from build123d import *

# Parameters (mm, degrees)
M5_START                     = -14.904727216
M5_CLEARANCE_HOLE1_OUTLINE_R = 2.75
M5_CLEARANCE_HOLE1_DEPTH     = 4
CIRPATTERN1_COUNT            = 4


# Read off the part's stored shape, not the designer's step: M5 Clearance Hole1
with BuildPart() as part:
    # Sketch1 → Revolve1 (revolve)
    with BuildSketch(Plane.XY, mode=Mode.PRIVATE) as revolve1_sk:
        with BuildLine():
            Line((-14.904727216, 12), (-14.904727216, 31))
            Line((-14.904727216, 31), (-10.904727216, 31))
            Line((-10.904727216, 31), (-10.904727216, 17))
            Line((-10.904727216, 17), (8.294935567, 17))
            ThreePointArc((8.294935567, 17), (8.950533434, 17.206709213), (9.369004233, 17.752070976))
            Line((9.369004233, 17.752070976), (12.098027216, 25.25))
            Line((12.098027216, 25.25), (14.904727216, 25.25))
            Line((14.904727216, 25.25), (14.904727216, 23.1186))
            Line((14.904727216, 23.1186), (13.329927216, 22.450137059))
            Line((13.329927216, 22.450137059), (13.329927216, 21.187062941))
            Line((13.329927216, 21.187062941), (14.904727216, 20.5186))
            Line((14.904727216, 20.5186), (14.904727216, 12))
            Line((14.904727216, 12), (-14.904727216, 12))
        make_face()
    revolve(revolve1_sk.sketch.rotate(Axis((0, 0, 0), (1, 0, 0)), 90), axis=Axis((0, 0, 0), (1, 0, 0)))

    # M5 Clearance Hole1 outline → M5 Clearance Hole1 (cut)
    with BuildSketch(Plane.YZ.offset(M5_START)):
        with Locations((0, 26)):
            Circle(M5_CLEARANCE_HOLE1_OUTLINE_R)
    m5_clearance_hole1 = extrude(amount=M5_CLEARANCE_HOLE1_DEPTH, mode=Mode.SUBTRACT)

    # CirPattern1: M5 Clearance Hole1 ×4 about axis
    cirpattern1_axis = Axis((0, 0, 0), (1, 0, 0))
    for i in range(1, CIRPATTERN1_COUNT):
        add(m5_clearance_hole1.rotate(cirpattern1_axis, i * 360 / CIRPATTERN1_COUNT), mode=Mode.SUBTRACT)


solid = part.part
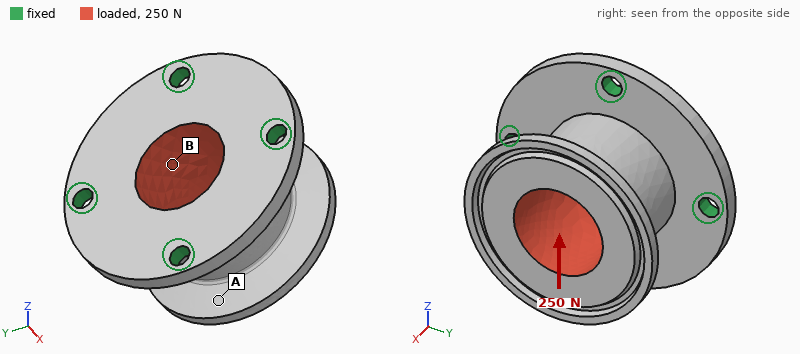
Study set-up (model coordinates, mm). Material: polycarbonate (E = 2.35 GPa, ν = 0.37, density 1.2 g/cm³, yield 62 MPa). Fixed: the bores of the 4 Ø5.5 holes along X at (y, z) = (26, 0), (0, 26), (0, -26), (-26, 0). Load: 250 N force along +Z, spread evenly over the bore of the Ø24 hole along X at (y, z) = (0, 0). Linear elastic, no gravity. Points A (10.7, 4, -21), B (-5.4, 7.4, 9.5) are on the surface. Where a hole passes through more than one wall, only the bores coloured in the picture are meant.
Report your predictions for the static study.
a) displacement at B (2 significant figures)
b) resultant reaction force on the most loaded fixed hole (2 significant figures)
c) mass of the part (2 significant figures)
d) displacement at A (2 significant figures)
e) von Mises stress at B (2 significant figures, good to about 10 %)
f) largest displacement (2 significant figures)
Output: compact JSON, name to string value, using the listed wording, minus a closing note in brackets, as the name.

{"displacement at B": "27 µm", "resultant reaction force on the most loaded fixed hole": "110 N", "mass of the part": "31 g", "displacement at A": "74 µm", "von Mises stress at B": "1.1 MPa", "largest displacement": "86 µm"}
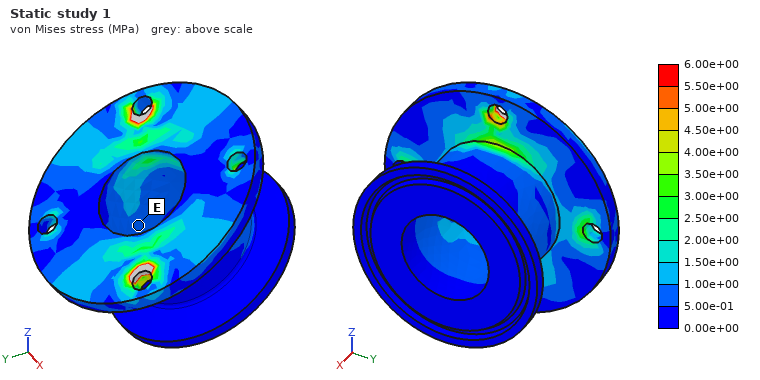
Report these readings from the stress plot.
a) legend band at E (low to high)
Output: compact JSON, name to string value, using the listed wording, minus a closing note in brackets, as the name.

{"legend band at E": "5.00e-01 to 1.00e+00 MPa"}
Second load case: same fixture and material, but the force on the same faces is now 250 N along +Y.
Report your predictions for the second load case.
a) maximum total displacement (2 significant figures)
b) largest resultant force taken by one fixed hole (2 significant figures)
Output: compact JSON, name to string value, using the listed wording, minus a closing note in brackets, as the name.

{"maximum total displacement": "86 µm", "largest resultant force taken by one fixed hole": "110 N"}
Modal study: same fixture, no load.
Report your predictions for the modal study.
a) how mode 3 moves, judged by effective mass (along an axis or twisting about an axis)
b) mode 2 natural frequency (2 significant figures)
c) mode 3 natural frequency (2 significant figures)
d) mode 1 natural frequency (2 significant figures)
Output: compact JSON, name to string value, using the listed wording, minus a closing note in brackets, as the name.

{"how mode 3 moves, judged by effective mass": "along X", "mode 2 natural frequency": "1800 Hz", "mode 3 natural frequency": "2700 Hz", "mode 1 natural frequency": "1800 Hz"}
